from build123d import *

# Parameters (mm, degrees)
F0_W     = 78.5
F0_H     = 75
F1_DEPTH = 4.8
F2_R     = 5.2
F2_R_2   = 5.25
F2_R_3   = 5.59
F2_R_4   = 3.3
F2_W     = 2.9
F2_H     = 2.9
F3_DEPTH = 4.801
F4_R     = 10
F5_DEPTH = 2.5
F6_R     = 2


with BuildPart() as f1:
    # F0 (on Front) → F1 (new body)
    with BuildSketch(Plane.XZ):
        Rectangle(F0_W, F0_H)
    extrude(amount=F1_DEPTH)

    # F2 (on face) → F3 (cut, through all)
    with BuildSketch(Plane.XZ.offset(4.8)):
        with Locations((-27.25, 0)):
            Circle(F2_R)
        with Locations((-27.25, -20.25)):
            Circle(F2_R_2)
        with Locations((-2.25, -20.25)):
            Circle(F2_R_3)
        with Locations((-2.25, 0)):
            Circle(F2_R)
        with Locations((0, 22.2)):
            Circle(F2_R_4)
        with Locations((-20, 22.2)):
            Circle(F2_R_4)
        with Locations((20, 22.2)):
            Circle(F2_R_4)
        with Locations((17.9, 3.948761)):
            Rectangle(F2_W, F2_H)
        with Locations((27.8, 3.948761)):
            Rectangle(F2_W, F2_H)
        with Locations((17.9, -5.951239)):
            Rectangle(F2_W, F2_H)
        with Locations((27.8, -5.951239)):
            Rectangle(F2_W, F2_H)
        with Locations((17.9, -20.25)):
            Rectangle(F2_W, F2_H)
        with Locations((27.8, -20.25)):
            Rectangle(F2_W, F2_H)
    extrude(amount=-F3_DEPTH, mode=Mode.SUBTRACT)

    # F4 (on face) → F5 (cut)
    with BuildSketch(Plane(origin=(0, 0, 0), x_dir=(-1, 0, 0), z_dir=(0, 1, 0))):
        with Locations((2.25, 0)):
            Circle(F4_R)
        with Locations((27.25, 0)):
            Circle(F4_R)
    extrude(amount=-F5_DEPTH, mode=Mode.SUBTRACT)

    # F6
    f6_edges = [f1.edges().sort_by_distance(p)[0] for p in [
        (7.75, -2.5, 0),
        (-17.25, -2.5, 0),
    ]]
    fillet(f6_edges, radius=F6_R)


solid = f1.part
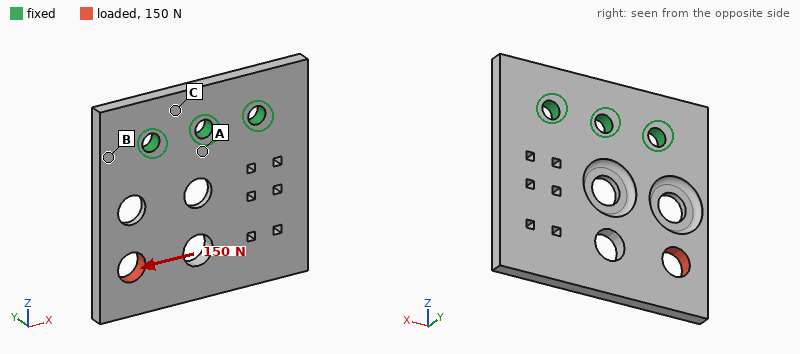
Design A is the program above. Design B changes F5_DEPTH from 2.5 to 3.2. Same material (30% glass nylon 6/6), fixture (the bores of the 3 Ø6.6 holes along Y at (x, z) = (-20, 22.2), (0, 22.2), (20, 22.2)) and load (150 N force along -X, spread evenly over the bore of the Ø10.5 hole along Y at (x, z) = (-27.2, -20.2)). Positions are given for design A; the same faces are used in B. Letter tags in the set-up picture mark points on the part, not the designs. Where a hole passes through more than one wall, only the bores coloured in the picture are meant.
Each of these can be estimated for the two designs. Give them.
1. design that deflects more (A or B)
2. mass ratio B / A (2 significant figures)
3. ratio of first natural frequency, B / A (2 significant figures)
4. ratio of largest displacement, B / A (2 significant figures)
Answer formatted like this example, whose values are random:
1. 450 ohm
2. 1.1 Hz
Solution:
1. B
2. 0.99
3. 0.99
4. 1.1
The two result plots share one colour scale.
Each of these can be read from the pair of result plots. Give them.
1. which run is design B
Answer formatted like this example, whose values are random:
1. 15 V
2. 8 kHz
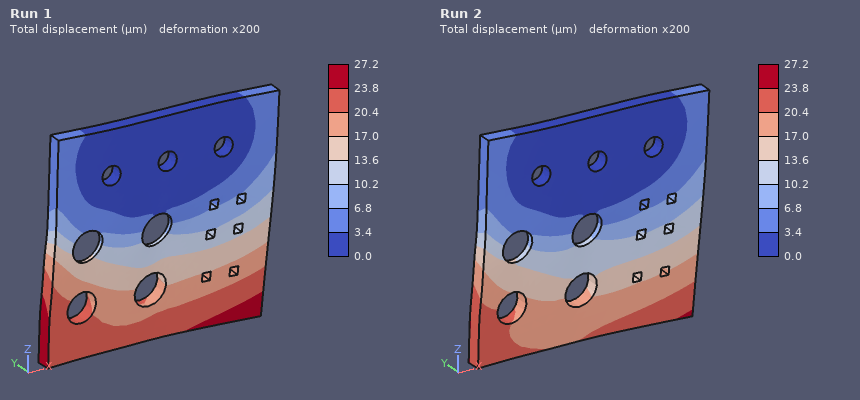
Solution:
1. Run 1
